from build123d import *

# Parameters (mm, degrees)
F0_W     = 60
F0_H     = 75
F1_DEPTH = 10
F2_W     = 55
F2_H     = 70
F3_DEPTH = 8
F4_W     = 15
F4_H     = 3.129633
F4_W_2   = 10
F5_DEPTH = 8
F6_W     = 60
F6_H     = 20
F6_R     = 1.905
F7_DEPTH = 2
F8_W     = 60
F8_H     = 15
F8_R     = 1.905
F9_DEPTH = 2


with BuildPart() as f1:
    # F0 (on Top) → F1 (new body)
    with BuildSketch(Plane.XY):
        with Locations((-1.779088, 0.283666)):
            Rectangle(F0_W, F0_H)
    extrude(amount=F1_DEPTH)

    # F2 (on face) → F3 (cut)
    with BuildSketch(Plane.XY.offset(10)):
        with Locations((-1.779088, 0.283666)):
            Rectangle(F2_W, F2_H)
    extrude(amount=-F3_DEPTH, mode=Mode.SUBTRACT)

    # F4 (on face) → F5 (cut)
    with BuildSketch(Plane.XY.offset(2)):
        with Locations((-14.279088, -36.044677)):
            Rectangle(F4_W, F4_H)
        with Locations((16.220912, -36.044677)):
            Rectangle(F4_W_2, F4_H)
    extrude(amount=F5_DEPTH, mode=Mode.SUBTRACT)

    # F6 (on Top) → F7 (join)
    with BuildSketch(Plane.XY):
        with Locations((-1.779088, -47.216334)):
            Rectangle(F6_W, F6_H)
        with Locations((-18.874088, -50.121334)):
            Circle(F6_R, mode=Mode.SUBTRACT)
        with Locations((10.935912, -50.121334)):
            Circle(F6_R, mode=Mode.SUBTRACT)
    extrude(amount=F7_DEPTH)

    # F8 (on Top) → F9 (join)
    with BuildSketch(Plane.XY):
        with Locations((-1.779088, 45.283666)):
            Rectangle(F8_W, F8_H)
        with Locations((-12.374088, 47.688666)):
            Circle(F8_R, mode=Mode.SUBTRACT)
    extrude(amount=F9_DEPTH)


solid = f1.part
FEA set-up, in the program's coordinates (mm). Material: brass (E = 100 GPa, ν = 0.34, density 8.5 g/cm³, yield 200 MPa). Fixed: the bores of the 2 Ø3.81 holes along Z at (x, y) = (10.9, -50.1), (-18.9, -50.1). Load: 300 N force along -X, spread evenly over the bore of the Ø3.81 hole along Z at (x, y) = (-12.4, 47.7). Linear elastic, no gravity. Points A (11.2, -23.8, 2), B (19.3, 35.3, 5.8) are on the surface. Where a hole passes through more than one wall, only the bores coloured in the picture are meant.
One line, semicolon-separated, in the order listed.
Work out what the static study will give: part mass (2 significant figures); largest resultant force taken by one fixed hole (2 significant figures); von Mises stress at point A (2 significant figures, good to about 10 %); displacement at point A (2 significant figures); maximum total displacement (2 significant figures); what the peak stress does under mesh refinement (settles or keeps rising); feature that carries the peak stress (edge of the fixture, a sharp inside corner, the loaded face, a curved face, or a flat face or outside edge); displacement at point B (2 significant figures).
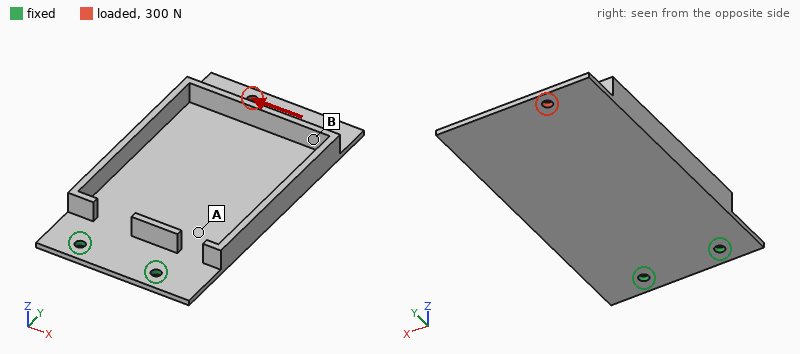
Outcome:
150 g; 930 N; 9.5 MPa; 13 µm; 57 µm; keeps rising; edge of the fixture; 45 µm
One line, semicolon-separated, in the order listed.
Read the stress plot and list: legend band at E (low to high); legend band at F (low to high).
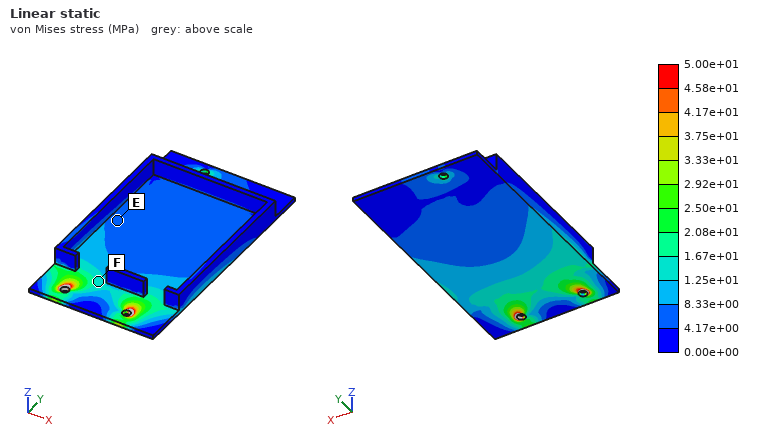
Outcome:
4.17e+00 to 8.33e+00 MPa; 1.25e+01 to 1.67e+01 MPa
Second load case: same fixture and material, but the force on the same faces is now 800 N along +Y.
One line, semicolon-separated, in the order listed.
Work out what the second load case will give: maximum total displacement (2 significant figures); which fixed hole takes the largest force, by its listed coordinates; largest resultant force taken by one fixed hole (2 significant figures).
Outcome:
40 µm; (-18.9, -50.1); 610 N
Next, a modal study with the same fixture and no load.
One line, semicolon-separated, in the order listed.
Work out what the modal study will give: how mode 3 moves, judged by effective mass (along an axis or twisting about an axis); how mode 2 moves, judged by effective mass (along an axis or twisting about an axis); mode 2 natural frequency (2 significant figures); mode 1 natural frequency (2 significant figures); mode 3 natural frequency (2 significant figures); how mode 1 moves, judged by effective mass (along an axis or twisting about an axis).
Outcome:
along Z; twisting about Y; 370 Hz; 120 Hz; 1400 Hz; along Z
